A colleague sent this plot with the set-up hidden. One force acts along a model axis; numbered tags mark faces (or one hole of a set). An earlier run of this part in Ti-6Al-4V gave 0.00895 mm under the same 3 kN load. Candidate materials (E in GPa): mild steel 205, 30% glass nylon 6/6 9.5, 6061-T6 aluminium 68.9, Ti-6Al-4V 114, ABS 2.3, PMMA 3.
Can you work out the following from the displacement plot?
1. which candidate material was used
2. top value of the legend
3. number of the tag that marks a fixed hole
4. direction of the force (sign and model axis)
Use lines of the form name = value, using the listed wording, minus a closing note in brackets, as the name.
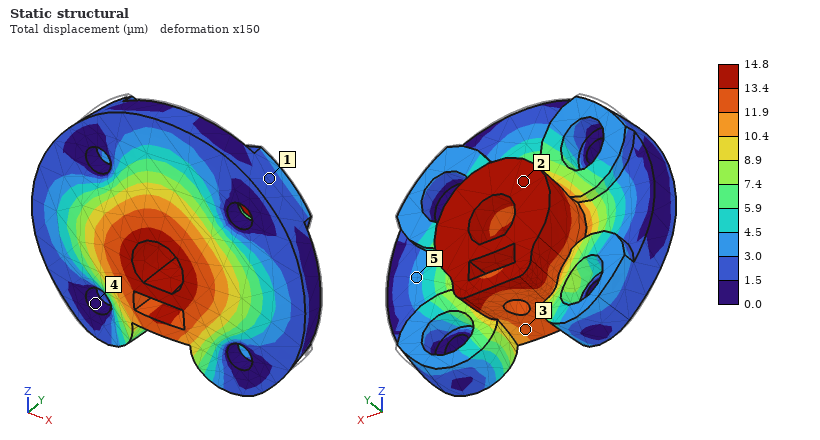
which candidate material was used = 6061-T6 aluminium
top value of the legend = 14.8 µm
number of the tag that marks a fixed hole = 4
direction of the force = -Y
